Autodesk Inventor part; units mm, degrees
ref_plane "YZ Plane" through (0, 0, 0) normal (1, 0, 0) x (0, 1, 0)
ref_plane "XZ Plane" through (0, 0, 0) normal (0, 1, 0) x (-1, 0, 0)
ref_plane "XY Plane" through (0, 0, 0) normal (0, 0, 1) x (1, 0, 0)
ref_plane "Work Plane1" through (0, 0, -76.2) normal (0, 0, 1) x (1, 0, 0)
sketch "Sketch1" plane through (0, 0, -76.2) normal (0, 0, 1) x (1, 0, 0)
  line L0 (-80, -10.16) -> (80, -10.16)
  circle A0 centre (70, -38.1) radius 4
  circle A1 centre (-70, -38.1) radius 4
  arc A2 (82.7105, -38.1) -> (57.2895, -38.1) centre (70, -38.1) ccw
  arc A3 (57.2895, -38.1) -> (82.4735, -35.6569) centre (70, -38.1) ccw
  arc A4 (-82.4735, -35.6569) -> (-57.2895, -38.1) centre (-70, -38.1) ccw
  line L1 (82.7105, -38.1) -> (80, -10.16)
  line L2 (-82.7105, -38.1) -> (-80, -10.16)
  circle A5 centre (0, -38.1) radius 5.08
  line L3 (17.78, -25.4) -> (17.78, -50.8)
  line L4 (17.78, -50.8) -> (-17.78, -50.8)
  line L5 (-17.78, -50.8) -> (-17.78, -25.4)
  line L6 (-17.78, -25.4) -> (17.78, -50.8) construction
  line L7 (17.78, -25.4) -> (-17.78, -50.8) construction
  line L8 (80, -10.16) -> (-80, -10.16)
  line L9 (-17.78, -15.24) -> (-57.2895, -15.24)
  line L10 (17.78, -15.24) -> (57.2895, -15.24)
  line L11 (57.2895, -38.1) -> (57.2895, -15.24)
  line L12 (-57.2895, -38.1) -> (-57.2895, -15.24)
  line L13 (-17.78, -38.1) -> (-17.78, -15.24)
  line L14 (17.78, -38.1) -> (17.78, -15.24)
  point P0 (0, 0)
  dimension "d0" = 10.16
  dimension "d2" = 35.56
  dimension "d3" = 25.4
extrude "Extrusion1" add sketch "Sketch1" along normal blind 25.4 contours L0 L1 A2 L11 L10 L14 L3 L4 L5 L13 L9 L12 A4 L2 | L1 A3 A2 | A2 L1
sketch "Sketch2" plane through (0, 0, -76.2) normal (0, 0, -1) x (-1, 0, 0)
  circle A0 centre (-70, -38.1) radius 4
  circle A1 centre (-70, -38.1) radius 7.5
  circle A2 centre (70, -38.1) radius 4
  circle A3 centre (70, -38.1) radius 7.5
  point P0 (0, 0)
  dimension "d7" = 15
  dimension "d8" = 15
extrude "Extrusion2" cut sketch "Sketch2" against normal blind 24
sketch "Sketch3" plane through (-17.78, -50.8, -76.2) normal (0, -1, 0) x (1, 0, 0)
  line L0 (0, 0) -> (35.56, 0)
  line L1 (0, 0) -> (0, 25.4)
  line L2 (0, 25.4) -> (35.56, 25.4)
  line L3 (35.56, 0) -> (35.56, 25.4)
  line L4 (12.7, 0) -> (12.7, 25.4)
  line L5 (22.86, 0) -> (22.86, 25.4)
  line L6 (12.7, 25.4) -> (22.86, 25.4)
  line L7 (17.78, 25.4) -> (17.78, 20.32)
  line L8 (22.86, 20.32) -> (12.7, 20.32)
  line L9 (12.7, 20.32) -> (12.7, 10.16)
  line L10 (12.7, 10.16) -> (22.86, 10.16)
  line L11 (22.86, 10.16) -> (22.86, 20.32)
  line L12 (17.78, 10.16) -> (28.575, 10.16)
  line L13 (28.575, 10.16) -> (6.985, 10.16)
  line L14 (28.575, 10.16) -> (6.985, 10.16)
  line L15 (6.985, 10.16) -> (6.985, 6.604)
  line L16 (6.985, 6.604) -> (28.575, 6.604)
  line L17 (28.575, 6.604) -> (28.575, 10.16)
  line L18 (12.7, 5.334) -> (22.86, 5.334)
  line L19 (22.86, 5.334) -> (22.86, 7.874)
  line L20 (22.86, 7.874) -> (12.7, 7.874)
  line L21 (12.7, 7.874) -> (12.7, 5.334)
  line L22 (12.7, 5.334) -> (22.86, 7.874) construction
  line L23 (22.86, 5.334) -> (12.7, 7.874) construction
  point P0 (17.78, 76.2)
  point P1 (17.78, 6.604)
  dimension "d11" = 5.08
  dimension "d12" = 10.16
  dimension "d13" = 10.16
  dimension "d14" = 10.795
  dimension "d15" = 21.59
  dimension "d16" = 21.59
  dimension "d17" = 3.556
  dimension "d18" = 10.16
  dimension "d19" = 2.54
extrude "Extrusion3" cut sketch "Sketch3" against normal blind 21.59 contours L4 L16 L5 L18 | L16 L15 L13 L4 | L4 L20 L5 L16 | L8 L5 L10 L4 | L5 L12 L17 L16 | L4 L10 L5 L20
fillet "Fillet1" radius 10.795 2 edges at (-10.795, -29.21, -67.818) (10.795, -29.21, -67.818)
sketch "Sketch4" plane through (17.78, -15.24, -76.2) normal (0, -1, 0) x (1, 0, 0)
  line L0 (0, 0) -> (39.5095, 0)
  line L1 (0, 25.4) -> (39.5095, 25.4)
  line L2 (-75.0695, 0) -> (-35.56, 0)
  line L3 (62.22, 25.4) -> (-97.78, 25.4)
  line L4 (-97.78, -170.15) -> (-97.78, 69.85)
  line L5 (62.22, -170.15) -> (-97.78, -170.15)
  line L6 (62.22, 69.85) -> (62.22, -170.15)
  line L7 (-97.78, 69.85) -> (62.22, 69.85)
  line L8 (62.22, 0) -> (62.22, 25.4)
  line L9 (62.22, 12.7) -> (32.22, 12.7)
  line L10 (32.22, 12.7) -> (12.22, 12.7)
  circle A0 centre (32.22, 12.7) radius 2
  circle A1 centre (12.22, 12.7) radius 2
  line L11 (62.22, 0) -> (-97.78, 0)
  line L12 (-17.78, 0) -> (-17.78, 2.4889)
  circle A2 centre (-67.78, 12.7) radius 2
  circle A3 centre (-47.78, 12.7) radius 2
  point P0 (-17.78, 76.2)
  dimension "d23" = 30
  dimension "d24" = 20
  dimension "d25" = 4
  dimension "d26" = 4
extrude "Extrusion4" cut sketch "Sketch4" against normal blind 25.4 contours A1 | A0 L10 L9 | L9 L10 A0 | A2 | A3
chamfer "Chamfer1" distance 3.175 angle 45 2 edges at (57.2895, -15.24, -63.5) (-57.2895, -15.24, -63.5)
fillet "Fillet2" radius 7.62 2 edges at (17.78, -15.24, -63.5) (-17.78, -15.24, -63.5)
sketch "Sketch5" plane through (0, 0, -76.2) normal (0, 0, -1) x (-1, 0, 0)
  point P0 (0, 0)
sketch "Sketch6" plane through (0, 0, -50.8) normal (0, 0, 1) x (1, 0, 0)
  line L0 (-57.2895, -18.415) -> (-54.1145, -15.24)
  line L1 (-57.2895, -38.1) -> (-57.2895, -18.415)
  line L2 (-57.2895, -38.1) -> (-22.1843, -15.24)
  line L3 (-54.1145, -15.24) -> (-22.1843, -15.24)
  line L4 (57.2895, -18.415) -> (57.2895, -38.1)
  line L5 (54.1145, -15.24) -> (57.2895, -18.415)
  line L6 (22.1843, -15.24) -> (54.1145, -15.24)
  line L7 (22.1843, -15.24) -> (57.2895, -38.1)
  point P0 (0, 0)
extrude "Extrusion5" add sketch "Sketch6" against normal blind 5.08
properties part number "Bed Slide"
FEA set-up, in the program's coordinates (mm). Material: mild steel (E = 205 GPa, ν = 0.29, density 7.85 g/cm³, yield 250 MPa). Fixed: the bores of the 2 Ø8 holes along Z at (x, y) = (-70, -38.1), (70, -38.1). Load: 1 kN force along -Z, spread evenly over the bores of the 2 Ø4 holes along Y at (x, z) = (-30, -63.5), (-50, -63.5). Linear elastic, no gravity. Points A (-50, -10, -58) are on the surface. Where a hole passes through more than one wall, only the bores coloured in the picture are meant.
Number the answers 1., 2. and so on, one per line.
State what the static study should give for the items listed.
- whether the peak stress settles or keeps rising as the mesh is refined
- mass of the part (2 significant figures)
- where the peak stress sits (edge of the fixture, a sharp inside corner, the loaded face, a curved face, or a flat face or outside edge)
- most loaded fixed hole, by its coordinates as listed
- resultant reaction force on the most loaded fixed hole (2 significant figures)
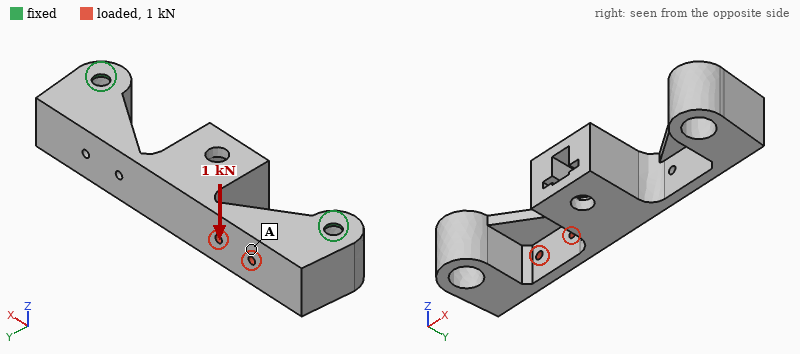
1. keeps rising
2. 670 g
3. edge of the fixture
4. (-70, -38.1)
5. 780 N
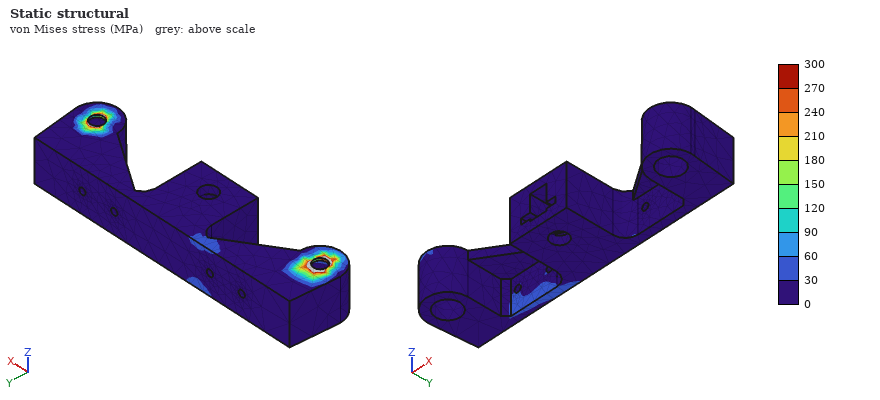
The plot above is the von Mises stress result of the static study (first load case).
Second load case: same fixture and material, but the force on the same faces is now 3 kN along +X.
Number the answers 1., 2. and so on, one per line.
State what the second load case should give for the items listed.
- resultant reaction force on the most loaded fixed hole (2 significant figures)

1. 1.6 kN
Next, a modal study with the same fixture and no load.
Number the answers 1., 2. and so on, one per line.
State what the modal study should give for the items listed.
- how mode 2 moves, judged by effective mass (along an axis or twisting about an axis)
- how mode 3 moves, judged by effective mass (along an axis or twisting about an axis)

1. along Z
2. along X
